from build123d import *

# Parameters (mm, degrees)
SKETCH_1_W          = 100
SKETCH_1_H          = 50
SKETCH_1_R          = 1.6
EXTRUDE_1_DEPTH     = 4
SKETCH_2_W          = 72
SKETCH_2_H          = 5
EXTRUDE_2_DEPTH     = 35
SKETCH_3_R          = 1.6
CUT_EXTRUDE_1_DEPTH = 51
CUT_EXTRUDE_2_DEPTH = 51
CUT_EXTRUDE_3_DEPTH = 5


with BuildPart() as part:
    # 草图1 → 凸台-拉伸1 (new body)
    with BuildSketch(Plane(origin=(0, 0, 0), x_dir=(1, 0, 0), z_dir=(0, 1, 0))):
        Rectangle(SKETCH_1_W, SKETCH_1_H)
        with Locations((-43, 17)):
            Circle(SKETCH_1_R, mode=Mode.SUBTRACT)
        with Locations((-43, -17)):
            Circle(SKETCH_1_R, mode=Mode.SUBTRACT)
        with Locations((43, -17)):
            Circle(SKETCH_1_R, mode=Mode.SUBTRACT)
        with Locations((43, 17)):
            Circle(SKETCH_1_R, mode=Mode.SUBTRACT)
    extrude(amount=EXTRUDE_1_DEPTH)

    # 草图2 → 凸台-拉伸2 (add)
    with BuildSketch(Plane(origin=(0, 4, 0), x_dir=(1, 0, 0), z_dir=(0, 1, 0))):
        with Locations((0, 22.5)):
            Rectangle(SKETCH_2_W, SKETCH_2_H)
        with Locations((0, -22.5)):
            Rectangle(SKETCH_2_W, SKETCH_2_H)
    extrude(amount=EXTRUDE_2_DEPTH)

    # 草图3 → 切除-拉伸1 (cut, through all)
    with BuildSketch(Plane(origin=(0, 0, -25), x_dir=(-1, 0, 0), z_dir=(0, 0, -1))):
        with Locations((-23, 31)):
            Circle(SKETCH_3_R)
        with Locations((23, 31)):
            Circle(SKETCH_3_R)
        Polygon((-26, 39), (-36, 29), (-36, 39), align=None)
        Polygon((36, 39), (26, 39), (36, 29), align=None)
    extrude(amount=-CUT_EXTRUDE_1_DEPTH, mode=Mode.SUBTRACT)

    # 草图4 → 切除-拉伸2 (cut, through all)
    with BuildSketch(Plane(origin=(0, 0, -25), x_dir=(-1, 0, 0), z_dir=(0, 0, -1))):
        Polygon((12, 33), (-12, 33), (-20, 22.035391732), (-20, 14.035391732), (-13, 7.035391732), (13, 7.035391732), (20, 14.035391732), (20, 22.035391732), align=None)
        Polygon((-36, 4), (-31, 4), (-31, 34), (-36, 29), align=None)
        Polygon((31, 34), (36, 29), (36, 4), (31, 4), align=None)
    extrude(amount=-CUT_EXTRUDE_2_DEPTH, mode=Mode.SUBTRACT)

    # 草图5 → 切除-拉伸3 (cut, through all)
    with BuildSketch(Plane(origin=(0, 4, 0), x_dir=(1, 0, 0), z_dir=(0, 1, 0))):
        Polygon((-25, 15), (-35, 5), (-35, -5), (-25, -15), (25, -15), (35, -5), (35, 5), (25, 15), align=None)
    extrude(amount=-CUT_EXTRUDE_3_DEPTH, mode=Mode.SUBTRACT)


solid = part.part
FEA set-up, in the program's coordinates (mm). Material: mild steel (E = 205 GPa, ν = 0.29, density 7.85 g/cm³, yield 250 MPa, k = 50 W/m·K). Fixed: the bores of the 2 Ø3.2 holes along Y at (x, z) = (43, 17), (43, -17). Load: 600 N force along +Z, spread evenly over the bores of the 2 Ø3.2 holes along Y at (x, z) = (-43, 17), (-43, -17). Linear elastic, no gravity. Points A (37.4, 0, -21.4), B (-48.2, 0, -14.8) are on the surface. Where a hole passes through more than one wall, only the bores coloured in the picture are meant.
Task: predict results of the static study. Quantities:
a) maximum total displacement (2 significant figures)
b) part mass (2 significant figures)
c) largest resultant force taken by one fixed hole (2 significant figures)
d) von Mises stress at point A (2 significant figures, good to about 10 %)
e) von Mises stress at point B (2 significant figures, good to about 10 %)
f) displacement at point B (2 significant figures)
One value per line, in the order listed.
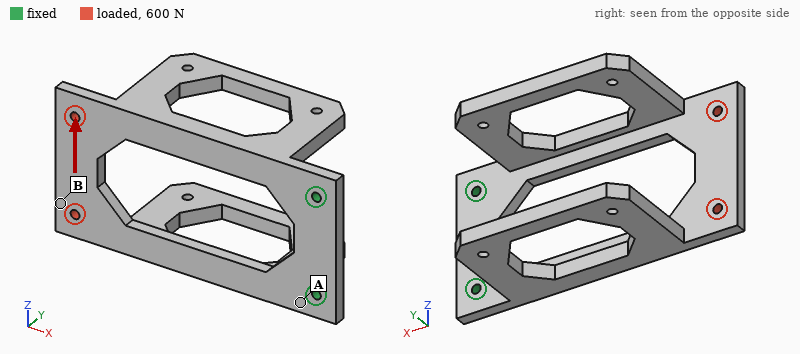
0.12 mm
190 g
1.4 kN
40 MPa
17 MPa
0.12 mm
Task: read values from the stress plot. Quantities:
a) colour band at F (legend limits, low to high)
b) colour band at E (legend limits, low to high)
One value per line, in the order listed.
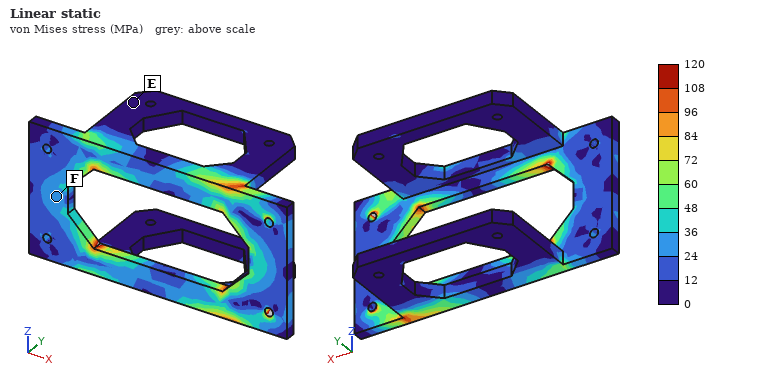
24 to 36 MPa
0 to 12 MPa
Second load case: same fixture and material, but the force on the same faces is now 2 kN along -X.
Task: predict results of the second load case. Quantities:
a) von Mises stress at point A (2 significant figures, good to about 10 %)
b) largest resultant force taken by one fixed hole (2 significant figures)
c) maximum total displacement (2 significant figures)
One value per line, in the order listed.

24 MPa
1.0 kN
21 µm
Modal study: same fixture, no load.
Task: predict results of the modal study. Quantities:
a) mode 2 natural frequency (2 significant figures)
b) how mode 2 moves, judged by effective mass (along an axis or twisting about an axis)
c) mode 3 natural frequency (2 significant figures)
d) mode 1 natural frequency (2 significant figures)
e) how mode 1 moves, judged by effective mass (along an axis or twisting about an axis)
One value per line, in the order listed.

690 Hz
along Z
1200 Hz
340 Hz
along Y
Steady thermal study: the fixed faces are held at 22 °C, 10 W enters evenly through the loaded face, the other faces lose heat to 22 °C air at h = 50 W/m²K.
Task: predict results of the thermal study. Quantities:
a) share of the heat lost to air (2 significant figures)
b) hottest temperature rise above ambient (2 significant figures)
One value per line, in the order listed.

89 %
44 K
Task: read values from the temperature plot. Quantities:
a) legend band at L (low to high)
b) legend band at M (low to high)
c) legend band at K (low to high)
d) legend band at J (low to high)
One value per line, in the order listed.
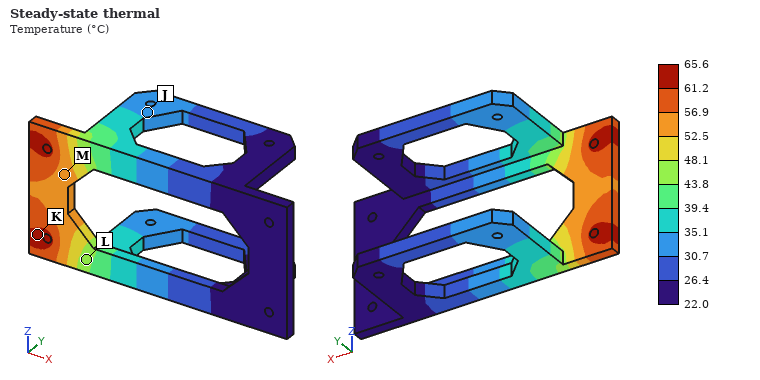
43.8 to 48.1 °C
52.5 to 56.9 °C
61.2 to 65.6 °C
30.7 to 35.1 °C
